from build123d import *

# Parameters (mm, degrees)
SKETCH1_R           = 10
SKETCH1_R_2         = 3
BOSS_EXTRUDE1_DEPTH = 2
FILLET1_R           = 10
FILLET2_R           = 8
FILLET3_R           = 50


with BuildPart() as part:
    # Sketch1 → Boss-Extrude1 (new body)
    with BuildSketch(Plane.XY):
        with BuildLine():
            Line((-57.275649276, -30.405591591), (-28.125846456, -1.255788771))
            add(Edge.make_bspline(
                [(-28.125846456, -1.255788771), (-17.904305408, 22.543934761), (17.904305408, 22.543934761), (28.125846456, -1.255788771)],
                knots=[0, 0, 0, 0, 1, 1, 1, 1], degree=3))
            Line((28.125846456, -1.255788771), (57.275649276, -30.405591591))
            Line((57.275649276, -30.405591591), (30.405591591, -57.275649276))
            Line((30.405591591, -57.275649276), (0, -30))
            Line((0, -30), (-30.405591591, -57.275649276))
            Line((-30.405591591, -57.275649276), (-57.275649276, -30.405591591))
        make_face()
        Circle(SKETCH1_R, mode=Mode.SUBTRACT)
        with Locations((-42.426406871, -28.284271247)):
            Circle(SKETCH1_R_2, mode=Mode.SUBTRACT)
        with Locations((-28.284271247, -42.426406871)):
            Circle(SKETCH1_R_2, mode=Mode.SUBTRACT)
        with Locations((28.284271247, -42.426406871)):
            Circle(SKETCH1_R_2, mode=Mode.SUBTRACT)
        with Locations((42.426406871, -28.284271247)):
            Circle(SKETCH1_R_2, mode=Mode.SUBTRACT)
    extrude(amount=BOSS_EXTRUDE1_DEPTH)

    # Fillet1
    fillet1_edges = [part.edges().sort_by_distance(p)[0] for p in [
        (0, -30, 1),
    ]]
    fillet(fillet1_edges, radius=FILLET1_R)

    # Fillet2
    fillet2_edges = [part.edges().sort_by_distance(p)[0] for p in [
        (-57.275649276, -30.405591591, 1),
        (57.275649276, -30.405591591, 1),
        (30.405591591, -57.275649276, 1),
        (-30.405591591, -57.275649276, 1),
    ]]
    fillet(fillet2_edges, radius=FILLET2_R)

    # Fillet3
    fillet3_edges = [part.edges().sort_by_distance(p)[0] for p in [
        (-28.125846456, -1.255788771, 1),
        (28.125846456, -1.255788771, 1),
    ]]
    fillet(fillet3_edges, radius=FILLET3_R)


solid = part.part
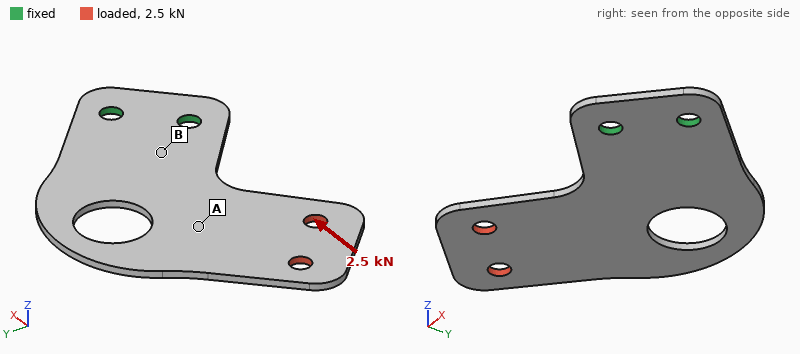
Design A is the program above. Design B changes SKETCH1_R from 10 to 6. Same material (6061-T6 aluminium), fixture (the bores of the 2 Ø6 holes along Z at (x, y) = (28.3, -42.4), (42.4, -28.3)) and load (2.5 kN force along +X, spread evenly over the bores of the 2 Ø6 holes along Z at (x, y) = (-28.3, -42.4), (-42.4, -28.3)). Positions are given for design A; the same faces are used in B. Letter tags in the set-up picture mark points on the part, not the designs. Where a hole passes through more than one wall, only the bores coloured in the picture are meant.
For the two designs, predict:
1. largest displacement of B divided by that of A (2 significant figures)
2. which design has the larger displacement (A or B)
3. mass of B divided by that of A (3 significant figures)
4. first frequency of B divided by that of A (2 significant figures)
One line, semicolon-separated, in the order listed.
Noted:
0.88; A; 1.05; 1.0
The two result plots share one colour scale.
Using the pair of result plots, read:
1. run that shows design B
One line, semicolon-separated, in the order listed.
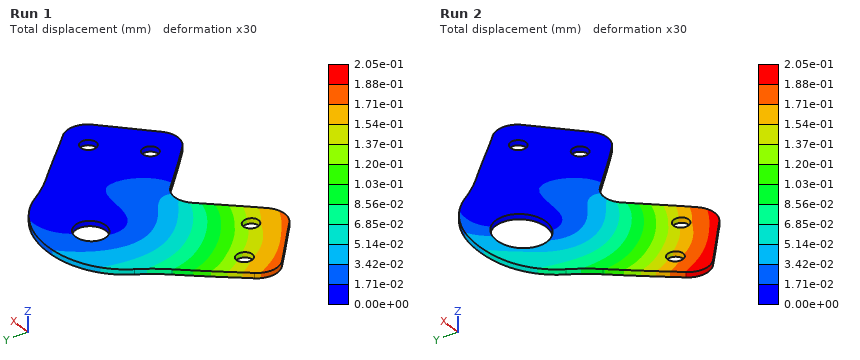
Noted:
Run 1
